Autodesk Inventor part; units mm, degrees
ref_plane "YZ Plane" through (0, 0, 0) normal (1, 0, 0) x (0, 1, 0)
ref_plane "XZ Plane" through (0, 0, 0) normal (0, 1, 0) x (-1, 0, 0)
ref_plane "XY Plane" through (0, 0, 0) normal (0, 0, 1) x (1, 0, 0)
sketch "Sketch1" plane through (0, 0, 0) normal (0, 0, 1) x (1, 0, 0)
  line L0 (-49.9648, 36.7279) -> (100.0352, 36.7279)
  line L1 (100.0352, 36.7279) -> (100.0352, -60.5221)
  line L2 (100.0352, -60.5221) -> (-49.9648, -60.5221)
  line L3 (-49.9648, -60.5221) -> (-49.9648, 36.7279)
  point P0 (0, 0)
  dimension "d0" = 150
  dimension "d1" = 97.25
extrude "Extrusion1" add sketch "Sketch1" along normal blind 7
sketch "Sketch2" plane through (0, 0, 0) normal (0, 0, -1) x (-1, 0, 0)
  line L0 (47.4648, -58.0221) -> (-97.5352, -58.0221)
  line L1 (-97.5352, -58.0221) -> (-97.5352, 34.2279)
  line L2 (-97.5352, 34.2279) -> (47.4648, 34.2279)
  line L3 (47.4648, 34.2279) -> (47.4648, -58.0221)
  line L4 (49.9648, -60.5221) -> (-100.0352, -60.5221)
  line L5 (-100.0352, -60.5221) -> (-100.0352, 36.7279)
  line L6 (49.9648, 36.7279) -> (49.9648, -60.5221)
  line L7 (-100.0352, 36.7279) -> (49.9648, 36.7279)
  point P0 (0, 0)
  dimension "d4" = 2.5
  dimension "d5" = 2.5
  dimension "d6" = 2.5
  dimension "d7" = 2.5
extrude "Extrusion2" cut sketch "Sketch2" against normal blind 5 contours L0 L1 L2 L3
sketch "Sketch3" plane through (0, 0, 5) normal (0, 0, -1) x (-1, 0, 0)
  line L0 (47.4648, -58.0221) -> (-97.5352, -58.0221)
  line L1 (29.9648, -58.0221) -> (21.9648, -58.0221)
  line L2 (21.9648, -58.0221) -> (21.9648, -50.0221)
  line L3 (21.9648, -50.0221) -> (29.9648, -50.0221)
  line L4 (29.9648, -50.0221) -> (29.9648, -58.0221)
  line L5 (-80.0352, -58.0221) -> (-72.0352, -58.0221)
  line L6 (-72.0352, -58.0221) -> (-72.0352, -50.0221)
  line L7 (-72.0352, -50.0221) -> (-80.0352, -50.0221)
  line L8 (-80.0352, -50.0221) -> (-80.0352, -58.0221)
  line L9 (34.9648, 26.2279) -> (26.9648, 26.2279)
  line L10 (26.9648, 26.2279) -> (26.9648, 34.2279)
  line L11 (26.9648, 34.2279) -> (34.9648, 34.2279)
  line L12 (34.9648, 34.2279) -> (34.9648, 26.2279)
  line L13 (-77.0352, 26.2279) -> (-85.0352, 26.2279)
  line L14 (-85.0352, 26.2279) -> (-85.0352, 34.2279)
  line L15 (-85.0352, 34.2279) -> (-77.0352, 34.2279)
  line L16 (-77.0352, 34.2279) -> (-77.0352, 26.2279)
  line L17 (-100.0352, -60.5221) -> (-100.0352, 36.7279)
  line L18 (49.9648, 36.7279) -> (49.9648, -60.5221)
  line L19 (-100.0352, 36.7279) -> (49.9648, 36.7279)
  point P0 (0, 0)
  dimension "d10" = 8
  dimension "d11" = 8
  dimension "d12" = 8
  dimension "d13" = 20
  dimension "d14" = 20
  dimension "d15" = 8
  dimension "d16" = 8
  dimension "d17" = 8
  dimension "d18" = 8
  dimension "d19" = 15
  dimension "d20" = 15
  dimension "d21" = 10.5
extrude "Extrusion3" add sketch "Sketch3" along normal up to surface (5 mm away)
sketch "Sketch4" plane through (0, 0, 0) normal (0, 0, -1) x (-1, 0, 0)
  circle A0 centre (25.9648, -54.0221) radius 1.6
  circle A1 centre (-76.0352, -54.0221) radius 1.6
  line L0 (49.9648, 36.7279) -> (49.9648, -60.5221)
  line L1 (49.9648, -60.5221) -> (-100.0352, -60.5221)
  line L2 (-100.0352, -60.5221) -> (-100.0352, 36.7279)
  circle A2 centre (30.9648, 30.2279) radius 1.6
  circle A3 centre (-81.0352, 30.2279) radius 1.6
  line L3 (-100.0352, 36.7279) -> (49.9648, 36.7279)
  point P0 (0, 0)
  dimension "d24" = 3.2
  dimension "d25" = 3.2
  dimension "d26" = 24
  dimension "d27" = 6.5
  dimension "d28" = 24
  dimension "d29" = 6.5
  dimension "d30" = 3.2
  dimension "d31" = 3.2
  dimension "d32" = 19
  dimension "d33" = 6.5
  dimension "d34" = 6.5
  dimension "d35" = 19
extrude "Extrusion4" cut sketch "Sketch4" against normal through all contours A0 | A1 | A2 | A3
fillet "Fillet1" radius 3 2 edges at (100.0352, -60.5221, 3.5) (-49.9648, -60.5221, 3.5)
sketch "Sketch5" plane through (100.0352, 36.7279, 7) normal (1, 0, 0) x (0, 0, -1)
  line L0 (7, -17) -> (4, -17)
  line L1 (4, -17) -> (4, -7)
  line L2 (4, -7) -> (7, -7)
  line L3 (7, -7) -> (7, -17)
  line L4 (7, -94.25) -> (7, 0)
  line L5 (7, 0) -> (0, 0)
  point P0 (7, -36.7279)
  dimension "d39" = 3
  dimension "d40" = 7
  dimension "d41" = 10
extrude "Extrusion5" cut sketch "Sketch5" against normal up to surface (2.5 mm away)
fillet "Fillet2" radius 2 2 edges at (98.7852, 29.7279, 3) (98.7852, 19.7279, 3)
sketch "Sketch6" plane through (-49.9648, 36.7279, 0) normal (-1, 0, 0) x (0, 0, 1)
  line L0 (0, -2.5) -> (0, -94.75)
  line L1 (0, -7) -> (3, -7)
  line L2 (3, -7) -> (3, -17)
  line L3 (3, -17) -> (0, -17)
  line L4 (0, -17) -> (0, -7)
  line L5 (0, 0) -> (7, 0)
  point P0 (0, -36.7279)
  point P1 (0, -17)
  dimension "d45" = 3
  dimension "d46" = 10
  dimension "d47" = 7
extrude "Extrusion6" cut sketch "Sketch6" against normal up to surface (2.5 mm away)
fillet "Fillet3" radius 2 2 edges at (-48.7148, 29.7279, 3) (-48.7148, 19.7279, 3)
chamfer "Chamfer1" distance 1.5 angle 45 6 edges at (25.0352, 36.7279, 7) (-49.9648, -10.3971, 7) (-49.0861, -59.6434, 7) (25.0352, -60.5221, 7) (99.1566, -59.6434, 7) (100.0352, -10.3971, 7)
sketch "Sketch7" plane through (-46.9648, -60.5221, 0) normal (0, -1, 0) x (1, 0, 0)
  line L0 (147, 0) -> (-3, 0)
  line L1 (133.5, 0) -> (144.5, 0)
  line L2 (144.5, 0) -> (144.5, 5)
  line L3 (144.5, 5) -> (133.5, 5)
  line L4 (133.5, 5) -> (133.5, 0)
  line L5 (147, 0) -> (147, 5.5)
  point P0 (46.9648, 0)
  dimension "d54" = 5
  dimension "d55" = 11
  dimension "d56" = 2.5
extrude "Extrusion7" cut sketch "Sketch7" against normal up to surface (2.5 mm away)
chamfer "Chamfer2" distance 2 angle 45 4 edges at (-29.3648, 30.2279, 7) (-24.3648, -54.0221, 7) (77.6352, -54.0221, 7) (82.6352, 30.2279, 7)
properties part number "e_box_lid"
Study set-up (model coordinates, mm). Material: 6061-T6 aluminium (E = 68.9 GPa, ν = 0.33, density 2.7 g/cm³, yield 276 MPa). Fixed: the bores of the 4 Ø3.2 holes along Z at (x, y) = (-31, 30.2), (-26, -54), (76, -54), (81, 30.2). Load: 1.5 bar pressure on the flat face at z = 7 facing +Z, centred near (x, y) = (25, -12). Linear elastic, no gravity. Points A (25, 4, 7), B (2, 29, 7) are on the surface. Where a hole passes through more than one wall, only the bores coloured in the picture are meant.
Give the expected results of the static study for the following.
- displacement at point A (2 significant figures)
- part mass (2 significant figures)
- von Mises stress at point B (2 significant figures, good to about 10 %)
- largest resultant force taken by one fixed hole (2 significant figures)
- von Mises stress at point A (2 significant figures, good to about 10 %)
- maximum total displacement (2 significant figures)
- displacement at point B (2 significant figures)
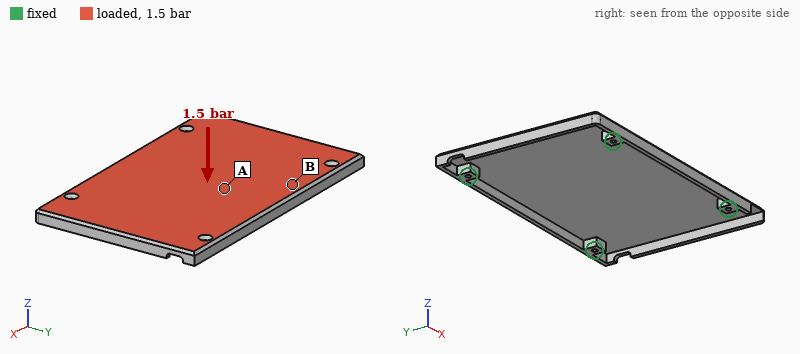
1.0 mm
95 g
39 MPa
800 N
91 MPa
1.1 mm
0.32 mm
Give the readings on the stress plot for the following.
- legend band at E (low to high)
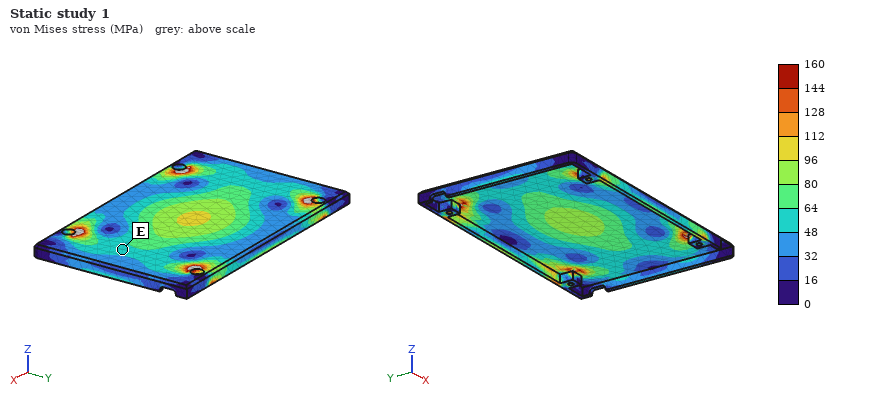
48 to 64 MPa
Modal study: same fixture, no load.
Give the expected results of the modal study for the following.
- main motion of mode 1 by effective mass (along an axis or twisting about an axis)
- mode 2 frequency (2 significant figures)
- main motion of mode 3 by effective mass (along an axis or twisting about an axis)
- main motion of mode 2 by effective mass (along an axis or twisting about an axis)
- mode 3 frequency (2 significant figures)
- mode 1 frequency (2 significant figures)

along Z
1800 Hz
along Z
twisting about Y
1900 Hz
990 Hz
